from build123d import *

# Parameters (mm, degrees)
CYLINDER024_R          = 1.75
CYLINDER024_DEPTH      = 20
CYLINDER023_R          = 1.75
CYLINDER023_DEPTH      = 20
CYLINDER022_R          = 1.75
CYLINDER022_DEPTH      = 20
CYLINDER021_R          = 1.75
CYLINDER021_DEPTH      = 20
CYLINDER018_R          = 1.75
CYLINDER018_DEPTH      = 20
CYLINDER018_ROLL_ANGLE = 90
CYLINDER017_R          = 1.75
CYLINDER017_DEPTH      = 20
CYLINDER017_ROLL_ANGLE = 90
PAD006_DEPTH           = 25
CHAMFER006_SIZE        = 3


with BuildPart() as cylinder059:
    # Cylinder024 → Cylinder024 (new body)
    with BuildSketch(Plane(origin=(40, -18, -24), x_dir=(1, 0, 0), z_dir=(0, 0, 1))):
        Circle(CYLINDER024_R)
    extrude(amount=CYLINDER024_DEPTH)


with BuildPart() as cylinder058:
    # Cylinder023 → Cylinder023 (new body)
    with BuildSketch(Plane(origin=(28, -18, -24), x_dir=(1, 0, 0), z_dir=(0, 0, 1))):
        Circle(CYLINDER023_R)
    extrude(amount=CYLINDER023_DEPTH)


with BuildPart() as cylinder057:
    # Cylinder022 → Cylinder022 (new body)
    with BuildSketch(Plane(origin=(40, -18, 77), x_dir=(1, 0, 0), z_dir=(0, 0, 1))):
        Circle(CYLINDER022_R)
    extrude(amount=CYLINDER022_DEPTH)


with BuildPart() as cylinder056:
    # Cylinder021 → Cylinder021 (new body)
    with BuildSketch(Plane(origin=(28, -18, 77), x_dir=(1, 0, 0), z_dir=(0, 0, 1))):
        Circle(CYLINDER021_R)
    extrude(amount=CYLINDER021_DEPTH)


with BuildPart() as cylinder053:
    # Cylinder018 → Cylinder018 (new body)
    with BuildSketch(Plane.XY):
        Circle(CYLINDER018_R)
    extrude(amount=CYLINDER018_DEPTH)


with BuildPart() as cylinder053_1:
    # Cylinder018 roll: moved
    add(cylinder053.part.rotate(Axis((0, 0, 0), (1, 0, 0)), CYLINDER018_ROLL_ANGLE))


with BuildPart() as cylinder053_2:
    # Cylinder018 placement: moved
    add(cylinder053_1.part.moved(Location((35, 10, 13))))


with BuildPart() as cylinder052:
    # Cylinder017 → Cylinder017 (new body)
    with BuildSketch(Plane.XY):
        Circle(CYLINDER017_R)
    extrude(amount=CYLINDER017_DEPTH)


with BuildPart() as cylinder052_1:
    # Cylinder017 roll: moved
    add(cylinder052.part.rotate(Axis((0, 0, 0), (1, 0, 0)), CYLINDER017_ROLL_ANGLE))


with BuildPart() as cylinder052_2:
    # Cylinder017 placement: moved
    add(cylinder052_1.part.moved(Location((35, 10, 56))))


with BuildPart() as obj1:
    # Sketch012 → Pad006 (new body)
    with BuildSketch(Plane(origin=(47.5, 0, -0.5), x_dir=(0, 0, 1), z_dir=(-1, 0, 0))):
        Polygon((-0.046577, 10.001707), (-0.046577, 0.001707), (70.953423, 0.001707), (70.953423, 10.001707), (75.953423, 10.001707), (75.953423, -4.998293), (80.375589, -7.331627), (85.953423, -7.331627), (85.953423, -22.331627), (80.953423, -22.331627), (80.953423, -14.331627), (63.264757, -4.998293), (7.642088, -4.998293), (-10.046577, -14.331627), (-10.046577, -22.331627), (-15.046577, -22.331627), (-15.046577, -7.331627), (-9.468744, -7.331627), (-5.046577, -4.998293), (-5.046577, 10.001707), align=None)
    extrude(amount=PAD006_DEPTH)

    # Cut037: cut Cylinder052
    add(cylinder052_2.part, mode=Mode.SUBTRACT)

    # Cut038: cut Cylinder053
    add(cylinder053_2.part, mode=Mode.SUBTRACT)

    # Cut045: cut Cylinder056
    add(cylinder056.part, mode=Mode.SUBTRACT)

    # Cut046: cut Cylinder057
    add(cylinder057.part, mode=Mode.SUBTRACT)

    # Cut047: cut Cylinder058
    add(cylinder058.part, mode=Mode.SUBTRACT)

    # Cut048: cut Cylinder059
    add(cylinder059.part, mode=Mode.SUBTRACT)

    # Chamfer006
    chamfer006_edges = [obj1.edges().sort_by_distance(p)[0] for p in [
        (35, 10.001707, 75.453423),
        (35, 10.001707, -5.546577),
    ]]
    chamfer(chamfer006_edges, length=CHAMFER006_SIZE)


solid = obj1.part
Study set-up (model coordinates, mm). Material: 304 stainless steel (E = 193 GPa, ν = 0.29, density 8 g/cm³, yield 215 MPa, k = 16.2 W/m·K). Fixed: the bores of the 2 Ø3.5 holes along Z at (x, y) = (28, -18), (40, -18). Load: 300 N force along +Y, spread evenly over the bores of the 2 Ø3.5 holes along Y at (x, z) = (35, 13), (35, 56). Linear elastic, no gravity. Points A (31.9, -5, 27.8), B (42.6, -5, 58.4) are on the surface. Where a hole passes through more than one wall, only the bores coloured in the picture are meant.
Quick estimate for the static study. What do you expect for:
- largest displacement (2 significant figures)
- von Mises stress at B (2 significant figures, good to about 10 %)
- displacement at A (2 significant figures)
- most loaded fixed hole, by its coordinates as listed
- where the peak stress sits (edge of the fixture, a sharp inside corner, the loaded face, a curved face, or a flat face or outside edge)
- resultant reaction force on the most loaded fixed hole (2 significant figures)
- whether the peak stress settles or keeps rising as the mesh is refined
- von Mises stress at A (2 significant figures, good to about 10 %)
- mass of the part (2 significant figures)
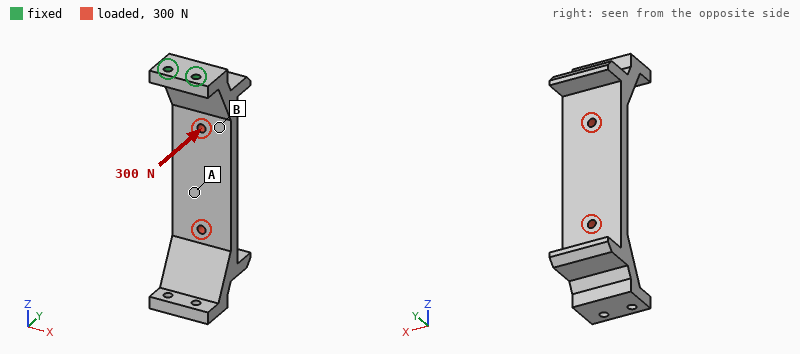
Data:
0.61 mm
71 MPa
0.26 mm
(40, -18)
edge of the fixture
190 N
keeps rising
22 MPa
160 g
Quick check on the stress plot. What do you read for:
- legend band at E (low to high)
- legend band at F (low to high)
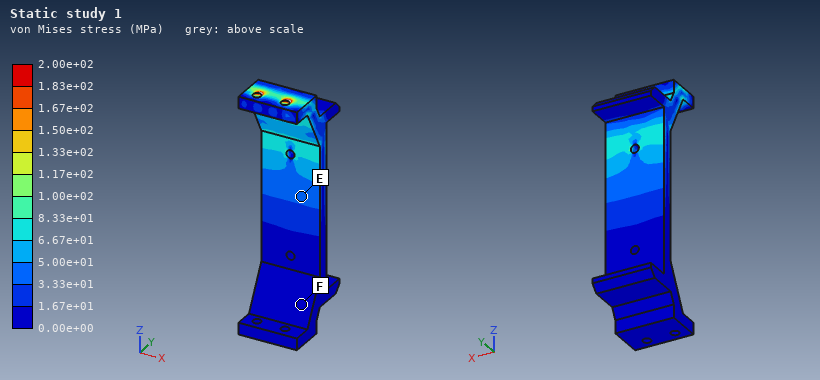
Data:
3.33e+01 to 5.00e+01 MPa
0.00e+00 to 1.67e+01 MPa
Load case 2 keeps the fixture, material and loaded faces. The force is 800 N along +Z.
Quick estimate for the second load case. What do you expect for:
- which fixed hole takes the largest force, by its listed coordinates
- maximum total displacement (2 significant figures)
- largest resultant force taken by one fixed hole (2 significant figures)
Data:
(40, -18)
0.17 mm
450 N
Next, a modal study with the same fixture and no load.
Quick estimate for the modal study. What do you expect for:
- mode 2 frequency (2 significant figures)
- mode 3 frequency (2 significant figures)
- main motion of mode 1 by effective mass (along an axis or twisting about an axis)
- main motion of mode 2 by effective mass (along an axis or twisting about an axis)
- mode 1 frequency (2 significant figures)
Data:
840 Hz
1800 Hz
along Y
along X
310 Hz
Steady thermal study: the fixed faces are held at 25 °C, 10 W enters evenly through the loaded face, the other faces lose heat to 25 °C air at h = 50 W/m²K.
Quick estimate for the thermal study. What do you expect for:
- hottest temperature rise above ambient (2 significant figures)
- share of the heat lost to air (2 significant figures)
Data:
45 K
84 %
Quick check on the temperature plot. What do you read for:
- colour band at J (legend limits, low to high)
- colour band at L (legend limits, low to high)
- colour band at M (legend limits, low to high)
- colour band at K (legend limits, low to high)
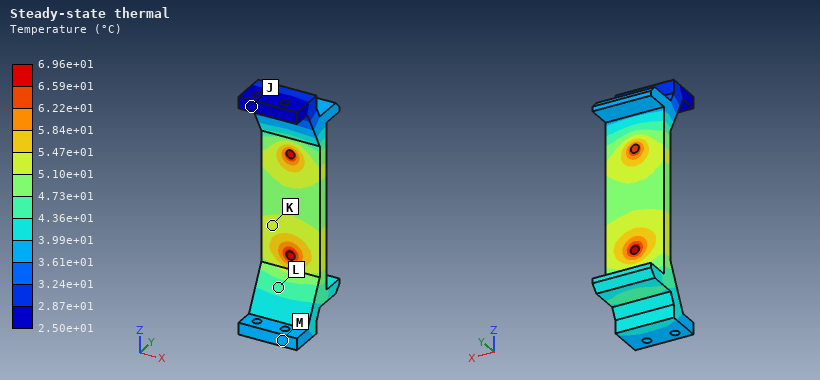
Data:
2.50e+01 to 2.87e+01 °C
4.36e+01 to 4.73e+01 °C
3.61e+01 to 3.99e+01 °C
5.10e+01 to 5.47e+01 °C
